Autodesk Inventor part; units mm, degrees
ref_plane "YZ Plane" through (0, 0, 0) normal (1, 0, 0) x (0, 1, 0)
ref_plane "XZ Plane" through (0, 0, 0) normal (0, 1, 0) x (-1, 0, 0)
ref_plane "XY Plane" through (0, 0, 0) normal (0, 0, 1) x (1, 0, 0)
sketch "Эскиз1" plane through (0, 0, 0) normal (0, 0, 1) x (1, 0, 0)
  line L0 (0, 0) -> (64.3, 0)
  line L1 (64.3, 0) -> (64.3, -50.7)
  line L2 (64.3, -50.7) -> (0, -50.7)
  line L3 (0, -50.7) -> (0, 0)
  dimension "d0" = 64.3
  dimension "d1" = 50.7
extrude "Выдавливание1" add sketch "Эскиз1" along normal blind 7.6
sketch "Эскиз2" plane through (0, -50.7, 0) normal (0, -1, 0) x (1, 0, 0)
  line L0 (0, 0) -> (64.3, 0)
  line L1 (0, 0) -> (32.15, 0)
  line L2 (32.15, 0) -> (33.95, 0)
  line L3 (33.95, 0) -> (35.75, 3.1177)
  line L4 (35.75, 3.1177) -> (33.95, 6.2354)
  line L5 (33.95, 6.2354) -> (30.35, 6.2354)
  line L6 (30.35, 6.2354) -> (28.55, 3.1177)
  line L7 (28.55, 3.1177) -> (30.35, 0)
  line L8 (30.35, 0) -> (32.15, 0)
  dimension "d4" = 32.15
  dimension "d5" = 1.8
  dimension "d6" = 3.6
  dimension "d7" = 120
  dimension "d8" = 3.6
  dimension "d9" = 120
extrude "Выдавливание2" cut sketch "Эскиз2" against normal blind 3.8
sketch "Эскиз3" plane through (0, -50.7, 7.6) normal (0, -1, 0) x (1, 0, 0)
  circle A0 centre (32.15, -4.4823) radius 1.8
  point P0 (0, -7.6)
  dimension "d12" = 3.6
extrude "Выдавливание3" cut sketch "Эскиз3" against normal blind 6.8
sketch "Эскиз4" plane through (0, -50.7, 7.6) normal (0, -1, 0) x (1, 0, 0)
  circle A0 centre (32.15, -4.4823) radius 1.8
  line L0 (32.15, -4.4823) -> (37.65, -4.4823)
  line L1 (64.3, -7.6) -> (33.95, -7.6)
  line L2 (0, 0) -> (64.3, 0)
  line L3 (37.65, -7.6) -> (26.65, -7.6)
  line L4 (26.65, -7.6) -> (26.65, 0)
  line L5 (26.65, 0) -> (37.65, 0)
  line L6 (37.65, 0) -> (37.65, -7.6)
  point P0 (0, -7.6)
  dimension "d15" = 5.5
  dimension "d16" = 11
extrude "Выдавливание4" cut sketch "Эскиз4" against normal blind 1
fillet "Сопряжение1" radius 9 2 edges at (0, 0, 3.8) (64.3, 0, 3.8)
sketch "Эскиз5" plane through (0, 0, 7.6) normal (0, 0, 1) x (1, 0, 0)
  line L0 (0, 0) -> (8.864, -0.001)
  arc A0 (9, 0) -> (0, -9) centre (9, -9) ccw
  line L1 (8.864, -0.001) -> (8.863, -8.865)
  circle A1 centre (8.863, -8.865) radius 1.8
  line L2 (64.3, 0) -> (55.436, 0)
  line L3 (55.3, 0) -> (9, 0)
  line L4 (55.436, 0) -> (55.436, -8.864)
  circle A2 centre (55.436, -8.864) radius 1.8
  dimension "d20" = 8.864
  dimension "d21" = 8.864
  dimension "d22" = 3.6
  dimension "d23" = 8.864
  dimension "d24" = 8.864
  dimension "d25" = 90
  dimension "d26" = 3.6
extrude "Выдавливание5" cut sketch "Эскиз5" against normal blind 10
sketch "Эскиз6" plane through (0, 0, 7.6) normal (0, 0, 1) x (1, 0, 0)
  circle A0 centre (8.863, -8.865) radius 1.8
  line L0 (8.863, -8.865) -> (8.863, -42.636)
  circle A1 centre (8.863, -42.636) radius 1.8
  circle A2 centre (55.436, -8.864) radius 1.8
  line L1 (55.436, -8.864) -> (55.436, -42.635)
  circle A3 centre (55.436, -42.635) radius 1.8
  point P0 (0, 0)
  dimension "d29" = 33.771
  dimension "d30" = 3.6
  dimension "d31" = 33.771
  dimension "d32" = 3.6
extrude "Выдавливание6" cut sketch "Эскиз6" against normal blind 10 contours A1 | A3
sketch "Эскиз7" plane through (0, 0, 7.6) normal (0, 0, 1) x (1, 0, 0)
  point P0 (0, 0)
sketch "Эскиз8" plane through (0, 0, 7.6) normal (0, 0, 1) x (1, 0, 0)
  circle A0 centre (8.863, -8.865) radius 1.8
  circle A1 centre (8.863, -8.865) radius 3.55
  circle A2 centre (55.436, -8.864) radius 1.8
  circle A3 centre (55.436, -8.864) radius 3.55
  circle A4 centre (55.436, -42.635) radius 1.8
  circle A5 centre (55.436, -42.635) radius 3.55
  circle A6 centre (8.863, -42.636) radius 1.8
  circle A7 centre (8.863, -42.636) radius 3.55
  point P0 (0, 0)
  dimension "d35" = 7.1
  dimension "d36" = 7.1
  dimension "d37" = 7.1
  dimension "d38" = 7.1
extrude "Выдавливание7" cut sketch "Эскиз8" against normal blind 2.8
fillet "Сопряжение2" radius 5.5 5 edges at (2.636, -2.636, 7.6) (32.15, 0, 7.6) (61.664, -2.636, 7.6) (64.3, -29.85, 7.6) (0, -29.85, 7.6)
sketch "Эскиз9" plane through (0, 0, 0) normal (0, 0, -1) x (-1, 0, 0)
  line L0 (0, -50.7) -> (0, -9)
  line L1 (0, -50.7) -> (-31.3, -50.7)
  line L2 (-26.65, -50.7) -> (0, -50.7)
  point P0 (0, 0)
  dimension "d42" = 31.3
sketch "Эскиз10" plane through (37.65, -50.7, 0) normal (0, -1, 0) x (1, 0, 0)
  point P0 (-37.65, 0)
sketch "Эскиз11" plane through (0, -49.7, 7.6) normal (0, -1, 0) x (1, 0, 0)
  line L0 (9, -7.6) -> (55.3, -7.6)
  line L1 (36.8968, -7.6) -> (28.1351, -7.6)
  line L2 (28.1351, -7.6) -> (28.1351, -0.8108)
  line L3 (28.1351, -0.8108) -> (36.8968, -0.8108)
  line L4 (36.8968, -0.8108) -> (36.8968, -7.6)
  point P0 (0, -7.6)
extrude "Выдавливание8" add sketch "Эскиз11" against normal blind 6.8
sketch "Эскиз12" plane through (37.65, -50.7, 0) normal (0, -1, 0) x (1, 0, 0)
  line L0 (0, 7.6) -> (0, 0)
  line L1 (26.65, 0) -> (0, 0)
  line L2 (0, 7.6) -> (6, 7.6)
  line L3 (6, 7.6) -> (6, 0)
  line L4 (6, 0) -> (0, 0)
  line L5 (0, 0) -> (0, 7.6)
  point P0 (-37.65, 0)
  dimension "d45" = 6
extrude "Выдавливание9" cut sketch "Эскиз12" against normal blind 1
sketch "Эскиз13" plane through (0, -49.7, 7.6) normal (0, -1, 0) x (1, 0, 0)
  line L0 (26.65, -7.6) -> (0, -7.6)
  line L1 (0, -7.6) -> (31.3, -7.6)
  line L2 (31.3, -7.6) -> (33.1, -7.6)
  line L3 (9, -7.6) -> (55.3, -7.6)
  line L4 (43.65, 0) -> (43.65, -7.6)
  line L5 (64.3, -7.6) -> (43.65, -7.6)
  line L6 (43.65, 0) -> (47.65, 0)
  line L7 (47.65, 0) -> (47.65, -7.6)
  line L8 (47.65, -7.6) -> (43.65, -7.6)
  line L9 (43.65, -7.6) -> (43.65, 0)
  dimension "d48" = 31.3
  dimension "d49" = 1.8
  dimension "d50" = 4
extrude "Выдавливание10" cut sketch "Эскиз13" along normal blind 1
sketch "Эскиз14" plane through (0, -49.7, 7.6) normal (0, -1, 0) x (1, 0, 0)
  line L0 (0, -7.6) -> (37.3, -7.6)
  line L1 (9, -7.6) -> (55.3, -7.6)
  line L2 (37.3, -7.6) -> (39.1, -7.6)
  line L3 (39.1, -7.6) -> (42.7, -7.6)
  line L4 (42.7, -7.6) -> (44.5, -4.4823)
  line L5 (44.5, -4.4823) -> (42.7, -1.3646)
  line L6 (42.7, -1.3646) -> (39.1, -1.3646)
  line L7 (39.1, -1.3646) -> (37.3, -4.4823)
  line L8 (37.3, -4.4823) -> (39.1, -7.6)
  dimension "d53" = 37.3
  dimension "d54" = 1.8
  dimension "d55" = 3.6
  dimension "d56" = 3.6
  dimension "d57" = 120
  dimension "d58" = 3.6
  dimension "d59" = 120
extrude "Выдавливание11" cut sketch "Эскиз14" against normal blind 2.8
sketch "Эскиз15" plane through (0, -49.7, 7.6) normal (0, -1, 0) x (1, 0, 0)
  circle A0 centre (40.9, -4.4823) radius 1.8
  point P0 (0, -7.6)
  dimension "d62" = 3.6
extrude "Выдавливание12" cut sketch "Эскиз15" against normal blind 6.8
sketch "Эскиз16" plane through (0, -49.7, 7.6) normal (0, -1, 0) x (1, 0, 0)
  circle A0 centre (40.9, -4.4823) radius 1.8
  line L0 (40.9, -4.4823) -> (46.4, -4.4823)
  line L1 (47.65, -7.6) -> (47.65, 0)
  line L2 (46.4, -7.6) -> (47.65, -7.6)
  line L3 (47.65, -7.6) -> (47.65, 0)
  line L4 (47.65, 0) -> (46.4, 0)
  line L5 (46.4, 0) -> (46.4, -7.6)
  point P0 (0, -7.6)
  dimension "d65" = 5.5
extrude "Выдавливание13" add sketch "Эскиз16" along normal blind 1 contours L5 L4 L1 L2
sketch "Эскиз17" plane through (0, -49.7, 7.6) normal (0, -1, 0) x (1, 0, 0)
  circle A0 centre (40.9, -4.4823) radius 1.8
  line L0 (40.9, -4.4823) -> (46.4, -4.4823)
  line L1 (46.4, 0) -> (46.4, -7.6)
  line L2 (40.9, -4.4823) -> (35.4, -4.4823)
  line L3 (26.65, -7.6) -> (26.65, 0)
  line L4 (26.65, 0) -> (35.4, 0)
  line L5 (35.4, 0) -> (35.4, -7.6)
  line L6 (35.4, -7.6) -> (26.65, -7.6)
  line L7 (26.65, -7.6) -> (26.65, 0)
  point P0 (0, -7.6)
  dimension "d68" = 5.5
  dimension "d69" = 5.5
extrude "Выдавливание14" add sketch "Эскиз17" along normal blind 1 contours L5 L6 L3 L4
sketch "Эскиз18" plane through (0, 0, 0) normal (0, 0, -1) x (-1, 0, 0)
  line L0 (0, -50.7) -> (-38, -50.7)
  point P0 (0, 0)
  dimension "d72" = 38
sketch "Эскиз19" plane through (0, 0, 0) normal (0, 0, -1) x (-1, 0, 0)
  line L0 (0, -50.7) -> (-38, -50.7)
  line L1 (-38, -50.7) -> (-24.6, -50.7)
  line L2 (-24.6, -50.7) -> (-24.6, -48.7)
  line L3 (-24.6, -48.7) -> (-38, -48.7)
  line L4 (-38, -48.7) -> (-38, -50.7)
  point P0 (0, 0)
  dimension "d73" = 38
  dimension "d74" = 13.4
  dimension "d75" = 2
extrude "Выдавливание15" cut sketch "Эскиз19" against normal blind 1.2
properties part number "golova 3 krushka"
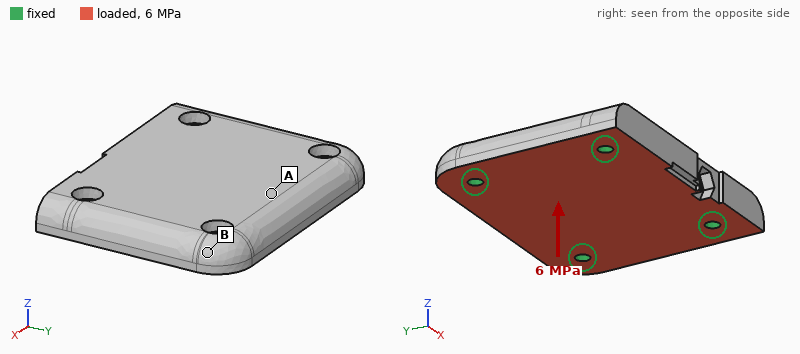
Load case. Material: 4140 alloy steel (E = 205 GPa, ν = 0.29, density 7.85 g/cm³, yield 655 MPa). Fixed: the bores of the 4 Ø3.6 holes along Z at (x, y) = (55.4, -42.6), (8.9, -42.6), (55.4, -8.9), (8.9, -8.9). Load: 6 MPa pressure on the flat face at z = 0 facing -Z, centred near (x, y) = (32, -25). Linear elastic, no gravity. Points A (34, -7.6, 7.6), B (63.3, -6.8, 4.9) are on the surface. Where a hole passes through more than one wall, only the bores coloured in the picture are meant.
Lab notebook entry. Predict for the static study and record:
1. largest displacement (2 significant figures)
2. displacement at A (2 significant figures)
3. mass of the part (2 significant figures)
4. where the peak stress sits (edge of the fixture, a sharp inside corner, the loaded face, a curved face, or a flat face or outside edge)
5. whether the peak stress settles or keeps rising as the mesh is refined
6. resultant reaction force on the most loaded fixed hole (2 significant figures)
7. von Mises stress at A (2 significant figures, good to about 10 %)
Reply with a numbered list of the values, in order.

1. 26 µm
2. 24 µm
3. 180 g
4. edge of the fixture
5. keeps rising
6. 5.1 kN
7. 98 MPa
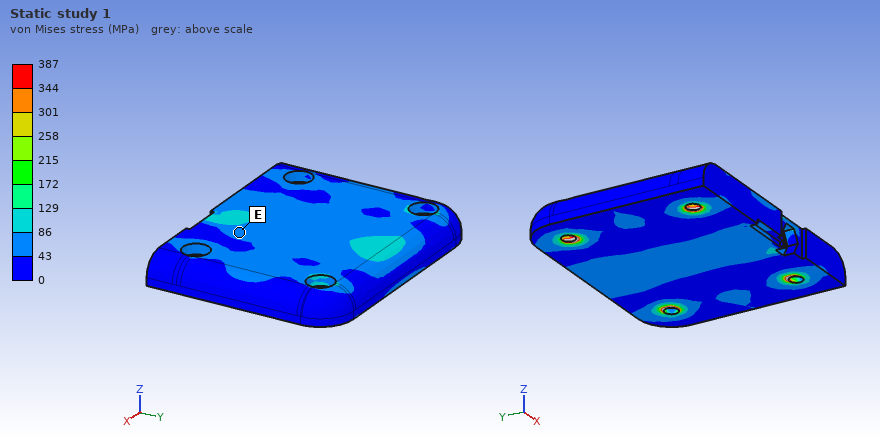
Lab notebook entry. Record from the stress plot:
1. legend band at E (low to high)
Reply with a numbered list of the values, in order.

1. 43 to 86 MPa
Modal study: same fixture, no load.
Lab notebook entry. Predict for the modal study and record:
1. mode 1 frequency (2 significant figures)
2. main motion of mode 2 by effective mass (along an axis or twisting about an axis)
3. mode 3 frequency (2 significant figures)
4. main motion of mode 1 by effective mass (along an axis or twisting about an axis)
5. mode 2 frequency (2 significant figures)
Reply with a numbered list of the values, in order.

1. 11 kHz
2. twisting about X
3. 19 kHz
4. along Z
5. 15 kHz
